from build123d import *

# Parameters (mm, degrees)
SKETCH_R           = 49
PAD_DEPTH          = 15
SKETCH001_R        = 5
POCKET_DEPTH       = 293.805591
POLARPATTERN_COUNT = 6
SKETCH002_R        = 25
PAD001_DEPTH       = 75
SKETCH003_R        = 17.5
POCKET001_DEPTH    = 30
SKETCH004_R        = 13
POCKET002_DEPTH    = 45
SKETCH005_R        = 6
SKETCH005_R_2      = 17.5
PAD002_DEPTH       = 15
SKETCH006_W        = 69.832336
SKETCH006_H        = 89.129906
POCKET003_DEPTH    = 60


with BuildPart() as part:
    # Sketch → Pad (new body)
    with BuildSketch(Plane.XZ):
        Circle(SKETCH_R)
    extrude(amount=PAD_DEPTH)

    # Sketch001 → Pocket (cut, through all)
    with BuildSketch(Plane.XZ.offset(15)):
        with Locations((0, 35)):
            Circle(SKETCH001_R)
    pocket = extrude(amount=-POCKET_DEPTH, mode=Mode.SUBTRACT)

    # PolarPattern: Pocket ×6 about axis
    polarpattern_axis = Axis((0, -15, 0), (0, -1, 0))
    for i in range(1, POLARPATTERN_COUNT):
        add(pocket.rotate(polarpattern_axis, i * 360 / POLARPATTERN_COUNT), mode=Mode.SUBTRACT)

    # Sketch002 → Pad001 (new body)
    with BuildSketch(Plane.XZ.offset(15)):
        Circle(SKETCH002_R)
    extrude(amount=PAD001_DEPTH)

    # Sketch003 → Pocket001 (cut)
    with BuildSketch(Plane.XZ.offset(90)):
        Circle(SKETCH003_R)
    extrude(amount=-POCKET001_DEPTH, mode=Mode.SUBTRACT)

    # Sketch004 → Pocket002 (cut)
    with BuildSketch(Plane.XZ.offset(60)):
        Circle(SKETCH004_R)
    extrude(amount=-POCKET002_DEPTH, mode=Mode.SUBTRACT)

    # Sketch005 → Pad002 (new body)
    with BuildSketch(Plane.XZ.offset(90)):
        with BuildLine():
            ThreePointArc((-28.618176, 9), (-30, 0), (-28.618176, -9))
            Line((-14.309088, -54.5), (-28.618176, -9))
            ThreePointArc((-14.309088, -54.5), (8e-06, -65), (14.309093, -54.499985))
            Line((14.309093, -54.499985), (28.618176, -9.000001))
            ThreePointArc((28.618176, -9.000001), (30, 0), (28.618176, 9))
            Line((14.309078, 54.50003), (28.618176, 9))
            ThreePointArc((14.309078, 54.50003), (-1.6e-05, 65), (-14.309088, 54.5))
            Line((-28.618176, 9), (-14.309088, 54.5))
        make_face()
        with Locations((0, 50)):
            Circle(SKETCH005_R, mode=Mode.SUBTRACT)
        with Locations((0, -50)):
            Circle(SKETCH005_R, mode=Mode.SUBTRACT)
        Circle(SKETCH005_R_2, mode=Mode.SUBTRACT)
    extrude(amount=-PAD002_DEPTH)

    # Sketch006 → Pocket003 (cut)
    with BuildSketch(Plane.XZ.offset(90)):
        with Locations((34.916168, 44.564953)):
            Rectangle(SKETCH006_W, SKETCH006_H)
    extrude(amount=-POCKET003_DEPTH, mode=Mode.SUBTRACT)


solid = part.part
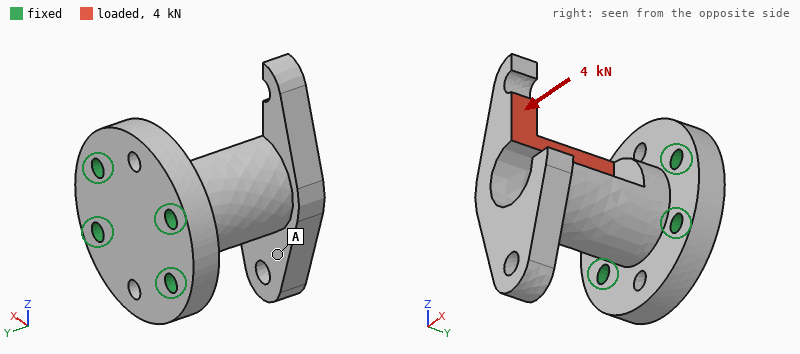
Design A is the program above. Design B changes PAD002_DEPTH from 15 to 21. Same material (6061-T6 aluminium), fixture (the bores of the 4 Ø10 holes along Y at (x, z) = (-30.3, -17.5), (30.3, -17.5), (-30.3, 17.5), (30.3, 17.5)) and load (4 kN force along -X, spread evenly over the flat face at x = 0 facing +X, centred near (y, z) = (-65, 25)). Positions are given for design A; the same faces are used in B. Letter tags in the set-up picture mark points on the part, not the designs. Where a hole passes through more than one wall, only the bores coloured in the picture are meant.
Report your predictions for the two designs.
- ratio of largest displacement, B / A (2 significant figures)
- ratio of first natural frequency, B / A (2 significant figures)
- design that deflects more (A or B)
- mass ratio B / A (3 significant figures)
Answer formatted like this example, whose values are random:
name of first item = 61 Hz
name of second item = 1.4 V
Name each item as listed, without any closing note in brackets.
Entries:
ratio of largest displacement, B / A = 0.91
ratio of first natural frequency, B / A = 0.95
design that deflects more = A
mass ratio B / A = 1.07
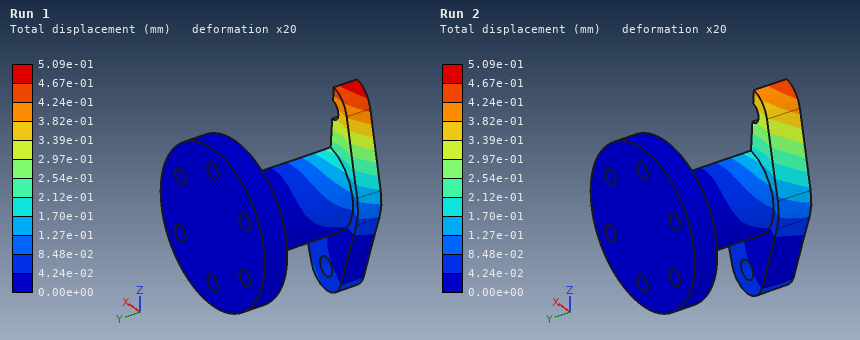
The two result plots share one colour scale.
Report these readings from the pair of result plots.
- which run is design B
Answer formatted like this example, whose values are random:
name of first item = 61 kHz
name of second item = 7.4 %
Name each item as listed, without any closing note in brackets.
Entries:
which run is design B = Run 2
